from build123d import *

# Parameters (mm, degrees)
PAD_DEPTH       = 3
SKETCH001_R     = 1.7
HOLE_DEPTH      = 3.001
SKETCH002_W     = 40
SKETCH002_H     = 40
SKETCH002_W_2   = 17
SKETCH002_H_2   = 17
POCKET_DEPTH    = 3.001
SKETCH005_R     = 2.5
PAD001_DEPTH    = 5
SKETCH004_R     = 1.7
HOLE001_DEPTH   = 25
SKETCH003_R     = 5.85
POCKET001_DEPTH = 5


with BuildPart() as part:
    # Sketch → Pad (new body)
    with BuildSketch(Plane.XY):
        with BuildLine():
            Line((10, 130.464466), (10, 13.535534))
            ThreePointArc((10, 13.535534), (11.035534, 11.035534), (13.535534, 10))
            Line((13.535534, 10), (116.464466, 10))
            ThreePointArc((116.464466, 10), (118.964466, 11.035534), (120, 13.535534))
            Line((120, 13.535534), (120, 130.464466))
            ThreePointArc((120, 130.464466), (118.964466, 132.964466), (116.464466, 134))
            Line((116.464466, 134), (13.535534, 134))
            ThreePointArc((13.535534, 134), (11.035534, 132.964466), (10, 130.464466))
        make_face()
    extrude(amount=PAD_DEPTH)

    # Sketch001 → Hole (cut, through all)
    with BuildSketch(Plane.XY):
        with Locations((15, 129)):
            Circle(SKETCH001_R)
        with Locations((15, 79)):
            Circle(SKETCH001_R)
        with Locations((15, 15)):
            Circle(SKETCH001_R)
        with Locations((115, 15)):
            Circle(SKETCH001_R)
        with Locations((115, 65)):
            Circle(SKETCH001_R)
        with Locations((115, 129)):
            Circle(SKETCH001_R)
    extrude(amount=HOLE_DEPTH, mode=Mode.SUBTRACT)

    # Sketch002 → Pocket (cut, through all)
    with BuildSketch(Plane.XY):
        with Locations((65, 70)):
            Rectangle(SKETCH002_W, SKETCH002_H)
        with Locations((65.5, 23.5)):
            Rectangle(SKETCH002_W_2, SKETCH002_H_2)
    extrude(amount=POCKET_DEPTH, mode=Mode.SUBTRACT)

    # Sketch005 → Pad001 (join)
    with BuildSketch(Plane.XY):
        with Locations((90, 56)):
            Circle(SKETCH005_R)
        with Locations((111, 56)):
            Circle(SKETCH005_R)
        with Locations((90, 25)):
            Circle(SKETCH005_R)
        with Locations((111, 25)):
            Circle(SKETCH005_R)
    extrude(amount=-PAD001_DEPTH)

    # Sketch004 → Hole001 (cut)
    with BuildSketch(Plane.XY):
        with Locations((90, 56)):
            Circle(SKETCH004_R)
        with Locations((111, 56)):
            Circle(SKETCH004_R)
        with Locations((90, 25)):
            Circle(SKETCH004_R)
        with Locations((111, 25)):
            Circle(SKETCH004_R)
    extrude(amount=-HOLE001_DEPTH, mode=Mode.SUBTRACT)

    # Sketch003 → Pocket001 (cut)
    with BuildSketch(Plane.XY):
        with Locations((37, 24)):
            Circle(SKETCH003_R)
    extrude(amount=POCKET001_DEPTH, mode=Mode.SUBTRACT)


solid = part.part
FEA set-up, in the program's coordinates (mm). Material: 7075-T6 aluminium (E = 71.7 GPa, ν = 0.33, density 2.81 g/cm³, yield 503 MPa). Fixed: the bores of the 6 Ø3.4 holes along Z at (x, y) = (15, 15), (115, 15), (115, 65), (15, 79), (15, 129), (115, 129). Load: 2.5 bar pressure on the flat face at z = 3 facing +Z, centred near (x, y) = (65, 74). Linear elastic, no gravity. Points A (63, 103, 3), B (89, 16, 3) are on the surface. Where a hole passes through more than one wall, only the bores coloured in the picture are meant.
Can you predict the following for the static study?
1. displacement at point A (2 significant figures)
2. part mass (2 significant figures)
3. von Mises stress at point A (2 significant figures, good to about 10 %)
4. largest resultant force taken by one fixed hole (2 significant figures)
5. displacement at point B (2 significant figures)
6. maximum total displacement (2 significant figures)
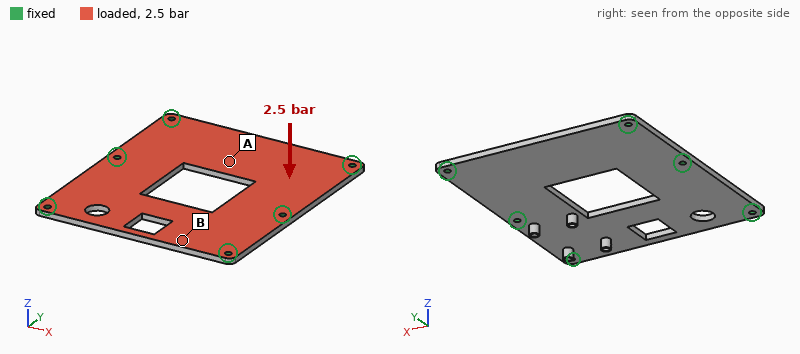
0.57 mm
98 g
74 MPa
680 N
0.32 mm
0.63 mm
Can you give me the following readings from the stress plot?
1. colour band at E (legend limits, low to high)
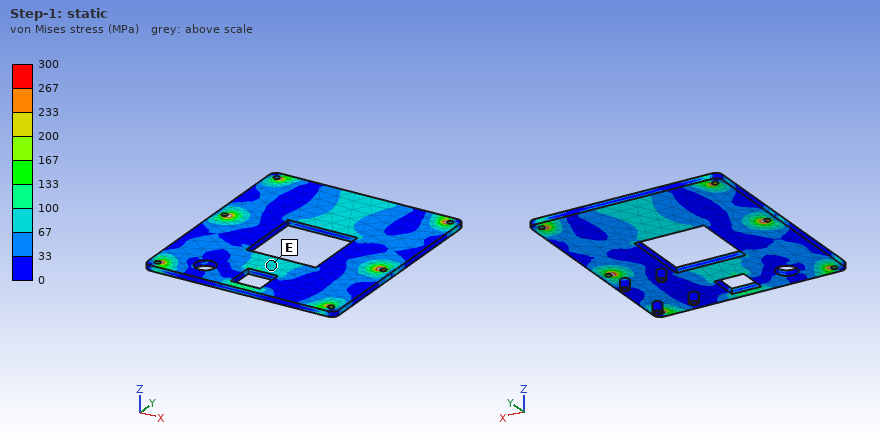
67 to 100 MPa
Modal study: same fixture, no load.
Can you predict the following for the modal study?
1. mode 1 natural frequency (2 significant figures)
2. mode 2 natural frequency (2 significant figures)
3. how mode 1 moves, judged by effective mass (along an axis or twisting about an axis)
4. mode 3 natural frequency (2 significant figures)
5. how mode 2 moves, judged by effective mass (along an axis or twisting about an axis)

1300 Hz
1500 Hz
along Z
2600 Hz
twisting about X
